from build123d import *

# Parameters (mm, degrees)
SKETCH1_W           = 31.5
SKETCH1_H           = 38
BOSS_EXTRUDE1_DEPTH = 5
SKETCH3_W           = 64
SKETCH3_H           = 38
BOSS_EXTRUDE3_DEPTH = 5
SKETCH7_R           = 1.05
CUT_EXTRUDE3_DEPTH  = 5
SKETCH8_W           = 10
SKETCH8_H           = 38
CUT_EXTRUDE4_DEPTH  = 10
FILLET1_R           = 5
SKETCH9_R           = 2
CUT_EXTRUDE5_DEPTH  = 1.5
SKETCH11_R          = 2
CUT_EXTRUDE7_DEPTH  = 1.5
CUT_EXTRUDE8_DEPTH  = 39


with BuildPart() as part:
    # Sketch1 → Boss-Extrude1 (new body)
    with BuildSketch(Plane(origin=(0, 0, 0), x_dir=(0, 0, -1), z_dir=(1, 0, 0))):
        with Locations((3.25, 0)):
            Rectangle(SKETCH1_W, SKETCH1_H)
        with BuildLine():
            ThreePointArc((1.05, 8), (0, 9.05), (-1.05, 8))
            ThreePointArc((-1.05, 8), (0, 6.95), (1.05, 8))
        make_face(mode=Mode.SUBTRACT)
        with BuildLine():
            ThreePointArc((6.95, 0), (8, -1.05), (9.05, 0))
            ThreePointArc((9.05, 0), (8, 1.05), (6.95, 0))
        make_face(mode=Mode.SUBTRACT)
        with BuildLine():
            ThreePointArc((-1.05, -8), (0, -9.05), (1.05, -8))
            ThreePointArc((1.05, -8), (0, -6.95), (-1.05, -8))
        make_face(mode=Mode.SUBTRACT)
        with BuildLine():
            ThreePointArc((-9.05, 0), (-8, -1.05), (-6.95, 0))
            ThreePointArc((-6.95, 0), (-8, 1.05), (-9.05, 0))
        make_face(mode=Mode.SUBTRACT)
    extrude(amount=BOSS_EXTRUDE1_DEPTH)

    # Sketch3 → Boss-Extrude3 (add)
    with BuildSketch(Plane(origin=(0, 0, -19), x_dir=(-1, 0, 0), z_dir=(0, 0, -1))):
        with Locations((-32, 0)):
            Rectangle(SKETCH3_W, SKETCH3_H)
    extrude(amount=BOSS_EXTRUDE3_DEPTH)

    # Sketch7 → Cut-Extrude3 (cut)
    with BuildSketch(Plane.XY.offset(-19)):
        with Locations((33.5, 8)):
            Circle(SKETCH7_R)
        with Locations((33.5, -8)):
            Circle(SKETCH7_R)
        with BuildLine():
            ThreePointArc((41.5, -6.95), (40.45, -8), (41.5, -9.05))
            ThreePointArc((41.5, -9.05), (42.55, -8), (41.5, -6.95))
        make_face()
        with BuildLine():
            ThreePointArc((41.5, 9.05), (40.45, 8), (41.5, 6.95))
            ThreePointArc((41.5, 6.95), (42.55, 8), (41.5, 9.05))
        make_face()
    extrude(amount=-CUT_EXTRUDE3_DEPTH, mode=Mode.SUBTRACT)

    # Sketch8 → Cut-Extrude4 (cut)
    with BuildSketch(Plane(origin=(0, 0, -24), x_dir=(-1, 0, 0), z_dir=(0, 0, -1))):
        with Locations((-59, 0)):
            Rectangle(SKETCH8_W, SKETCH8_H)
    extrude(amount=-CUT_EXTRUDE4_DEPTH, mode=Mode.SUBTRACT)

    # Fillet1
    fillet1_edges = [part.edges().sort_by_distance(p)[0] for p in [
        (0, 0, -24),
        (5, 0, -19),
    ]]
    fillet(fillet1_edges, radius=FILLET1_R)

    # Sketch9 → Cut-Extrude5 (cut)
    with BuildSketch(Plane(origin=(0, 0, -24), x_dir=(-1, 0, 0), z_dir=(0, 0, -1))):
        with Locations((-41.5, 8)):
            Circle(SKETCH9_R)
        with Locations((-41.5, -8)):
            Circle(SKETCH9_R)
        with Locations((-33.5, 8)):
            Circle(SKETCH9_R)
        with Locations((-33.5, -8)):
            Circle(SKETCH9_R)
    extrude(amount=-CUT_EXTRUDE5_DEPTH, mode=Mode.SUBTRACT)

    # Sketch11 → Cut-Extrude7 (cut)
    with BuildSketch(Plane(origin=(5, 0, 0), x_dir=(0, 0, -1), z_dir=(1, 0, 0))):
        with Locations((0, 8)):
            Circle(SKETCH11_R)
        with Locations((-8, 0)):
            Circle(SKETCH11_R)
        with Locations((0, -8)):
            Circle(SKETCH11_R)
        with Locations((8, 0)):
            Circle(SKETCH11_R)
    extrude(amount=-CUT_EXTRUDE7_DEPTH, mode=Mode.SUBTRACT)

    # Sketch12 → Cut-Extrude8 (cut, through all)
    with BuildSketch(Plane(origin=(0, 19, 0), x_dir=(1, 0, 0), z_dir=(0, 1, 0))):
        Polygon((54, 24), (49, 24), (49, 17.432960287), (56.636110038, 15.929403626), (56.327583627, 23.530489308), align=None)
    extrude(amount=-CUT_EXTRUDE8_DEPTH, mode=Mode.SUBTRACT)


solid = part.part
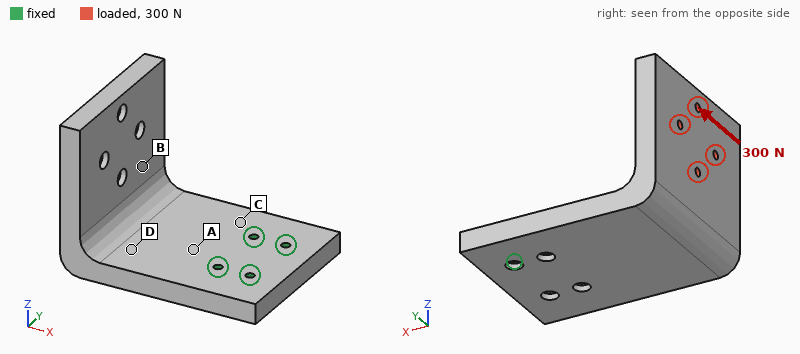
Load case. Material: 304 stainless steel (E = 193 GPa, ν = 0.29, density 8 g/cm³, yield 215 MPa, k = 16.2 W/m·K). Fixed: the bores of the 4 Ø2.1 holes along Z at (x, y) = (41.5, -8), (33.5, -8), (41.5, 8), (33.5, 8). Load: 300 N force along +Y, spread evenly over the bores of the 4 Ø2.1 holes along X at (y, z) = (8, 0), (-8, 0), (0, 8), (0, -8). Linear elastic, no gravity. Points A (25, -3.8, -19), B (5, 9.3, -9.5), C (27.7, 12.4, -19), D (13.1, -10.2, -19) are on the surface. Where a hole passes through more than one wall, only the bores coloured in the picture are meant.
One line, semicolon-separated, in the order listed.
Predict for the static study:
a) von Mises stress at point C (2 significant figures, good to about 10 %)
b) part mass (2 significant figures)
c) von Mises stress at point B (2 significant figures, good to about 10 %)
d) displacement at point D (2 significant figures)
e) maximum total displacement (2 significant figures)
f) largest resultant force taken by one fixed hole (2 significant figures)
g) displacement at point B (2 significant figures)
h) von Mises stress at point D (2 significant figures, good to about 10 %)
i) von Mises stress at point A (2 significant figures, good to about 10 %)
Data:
21 MPa; 120 g; 9.5 MPa; 9.9 µm; 50 µm; 540 N; 20 µm; 29 MPa; 34 MPa
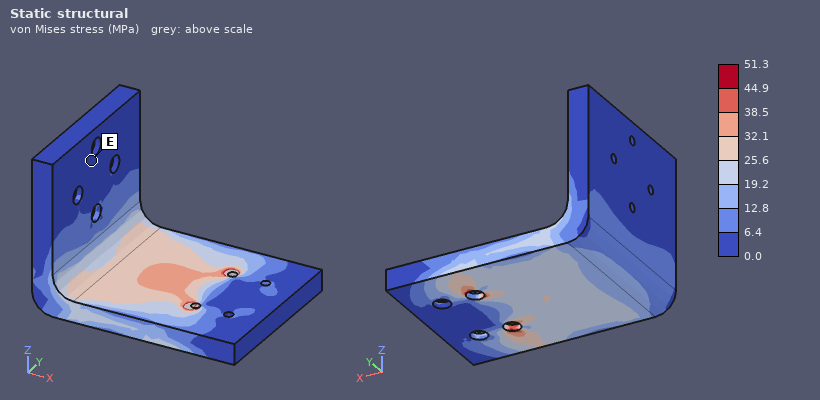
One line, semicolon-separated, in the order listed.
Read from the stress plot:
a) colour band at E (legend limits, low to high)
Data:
0.0 to 6.4 MPa
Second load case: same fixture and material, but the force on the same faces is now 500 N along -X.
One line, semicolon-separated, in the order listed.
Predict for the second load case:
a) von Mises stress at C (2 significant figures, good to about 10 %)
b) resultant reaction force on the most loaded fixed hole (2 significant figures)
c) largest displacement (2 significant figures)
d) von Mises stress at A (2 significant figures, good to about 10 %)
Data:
65 MPa; 530 N; 0.19 mm; 66 MPa
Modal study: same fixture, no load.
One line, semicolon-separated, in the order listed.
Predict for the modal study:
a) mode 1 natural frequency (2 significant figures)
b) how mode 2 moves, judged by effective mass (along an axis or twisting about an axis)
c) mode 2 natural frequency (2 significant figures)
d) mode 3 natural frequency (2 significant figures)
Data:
1200 Hz; along Y; 2100 Hz; 3700 Hz
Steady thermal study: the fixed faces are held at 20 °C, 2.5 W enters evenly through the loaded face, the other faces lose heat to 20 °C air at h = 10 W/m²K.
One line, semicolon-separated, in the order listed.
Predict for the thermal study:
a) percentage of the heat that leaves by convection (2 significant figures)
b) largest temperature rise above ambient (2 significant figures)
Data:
40 %; 32 K
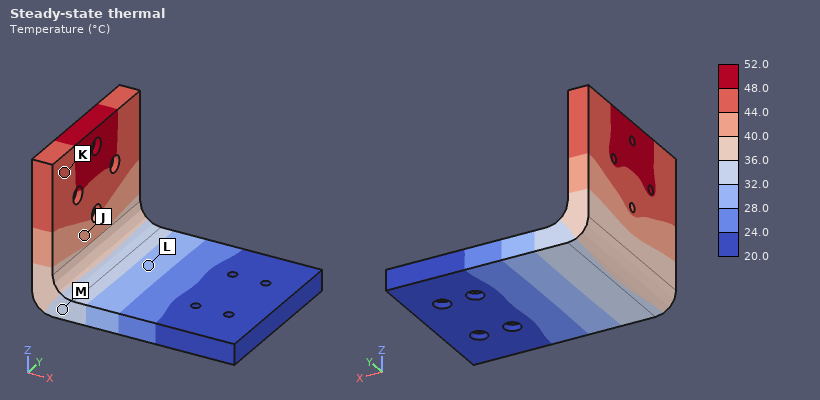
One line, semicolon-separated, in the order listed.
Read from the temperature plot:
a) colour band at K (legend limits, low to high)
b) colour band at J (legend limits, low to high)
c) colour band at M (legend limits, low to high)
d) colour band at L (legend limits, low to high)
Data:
44.0 to 48.0 °C; 40.0 to 44.0 °C; 32.0 to 36.0 °C; 28.0 to 32.0 °C
